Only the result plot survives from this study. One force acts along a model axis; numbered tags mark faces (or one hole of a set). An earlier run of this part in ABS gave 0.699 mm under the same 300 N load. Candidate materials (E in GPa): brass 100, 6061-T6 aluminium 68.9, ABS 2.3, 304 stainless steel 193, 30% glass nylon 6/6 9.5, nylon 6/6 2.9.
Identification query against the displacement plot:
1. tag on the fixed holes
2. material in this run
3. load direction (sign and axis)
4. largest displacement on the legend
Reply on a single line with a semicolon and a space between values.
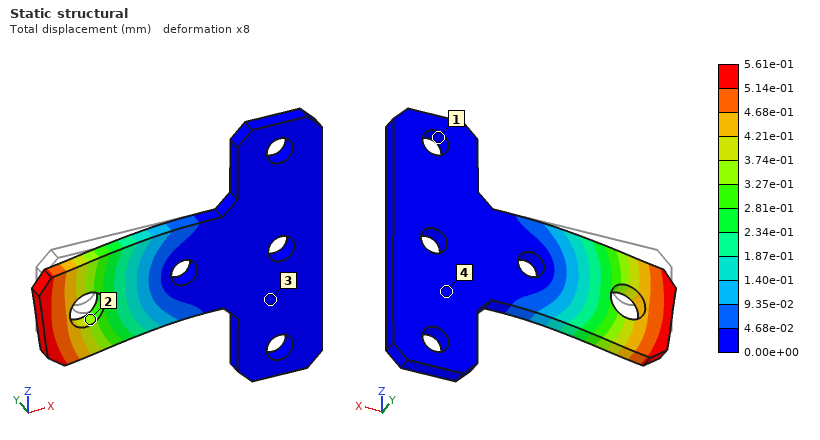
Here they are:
1; nylon 6/6; -Z; 5.61e-01 mm
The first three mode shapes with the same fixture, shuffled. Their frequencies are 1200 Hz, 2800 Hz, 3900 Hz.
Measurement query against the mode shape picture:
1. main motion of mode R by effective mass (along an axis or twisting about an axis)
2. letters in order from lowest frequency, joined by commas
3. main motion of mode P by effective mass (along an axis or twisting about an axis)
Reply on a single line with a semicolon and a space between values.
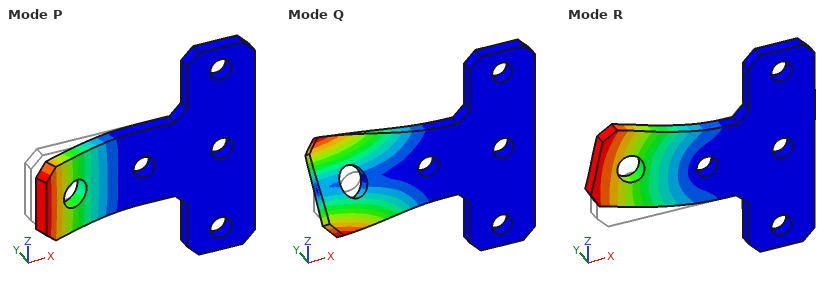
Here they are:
along Z; P, Q, R; along Y
